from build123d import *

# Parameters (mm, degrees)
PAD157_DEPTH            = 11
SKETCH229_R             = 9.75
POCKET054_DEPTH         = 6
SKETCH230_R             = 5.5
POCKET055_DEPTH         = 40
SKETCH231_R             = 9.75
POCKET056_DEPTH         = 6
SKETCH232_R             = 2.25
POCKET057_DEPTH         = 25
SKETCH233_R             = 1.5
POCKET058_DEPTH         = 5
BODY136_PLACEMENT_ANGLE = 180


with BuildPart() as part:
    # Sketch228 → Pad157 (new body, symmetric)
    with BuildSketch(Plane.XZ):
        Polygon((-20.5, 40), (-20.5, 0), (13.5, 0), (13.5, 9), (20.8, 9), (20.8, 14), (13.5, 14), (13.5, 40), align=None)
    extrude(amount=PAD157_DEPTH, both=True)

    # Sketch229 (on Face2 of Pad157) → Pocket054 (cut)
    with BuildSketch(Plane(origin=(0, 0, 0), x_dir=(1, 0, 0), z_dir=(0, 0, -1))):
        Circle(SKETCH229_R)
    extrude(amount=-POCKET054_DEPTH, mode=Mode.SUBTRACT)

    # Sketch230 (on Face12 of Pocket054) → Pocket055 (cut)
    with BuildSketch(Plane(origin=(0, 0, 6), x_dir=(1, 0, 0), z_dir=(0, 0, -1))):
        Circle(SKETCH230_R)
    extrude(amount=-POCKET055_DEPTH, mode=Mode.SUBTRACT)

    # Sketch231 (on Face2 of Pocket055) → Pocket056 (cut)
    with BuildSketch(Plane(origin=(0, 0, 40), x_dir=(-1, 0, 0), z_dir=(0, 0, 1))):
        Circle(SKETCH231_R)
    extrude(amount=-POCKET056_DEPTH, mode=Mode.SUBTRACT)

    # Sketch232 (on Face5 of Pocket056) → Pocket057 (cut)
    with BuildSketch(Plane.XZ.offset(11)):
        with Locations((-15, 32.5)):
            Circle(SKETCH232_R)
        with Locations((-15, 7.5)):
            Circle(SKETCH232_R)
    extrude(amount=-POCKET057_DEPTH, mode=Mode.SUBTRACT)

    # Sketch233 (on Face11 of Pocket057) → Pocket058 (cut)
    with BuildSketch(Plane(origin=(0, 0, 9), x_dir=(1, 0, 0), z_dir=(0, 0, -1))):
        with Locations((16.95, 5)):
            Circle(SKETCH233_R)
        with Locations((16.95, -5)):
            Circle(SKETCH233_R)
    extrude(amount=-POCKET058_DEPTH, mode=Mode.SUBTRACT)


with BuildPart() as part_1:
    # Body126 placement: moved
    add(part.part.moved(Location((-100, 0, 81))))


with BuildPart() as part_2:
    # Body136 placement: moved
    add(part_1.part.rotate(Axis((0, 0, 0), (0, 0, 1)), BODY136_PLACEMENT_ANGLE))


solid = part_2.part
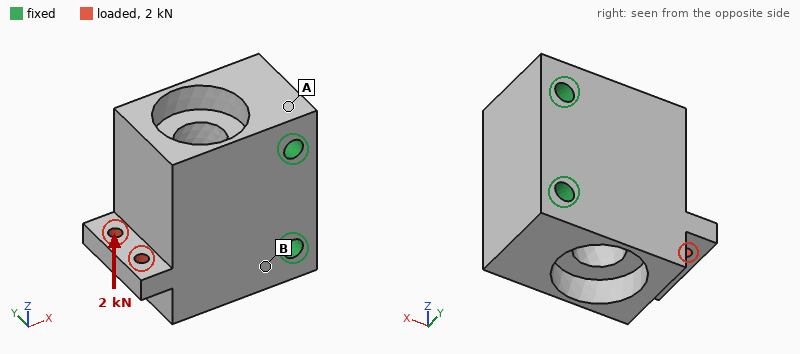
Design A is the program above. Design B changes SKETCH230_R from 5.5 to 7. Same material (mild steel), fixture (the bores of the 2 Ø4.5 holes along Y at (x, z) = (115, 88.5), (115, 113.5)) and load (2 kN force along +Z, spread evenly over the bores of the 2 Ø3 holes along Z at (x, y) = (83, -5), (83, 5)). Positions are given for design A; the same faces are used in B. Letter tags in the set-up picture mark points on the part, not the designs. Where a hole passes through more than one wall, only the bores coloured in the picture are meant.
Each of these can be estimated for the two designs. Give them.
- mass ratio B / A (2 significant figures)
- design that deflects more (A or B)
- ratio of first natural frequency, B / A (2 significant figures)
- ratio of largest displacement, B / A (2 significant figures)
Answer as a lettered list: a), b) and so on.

a) 0.93
b) B
c) 0.86
d) 1.1
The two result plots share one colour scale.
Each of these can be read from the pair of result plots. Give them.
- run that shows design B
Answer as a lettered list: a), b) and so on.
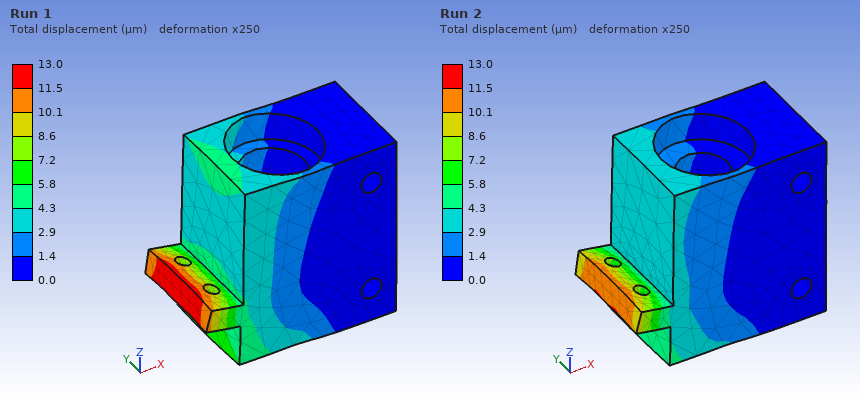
a) Run 1
